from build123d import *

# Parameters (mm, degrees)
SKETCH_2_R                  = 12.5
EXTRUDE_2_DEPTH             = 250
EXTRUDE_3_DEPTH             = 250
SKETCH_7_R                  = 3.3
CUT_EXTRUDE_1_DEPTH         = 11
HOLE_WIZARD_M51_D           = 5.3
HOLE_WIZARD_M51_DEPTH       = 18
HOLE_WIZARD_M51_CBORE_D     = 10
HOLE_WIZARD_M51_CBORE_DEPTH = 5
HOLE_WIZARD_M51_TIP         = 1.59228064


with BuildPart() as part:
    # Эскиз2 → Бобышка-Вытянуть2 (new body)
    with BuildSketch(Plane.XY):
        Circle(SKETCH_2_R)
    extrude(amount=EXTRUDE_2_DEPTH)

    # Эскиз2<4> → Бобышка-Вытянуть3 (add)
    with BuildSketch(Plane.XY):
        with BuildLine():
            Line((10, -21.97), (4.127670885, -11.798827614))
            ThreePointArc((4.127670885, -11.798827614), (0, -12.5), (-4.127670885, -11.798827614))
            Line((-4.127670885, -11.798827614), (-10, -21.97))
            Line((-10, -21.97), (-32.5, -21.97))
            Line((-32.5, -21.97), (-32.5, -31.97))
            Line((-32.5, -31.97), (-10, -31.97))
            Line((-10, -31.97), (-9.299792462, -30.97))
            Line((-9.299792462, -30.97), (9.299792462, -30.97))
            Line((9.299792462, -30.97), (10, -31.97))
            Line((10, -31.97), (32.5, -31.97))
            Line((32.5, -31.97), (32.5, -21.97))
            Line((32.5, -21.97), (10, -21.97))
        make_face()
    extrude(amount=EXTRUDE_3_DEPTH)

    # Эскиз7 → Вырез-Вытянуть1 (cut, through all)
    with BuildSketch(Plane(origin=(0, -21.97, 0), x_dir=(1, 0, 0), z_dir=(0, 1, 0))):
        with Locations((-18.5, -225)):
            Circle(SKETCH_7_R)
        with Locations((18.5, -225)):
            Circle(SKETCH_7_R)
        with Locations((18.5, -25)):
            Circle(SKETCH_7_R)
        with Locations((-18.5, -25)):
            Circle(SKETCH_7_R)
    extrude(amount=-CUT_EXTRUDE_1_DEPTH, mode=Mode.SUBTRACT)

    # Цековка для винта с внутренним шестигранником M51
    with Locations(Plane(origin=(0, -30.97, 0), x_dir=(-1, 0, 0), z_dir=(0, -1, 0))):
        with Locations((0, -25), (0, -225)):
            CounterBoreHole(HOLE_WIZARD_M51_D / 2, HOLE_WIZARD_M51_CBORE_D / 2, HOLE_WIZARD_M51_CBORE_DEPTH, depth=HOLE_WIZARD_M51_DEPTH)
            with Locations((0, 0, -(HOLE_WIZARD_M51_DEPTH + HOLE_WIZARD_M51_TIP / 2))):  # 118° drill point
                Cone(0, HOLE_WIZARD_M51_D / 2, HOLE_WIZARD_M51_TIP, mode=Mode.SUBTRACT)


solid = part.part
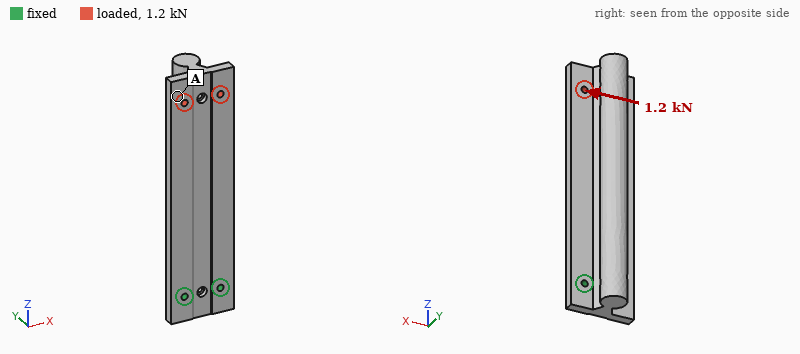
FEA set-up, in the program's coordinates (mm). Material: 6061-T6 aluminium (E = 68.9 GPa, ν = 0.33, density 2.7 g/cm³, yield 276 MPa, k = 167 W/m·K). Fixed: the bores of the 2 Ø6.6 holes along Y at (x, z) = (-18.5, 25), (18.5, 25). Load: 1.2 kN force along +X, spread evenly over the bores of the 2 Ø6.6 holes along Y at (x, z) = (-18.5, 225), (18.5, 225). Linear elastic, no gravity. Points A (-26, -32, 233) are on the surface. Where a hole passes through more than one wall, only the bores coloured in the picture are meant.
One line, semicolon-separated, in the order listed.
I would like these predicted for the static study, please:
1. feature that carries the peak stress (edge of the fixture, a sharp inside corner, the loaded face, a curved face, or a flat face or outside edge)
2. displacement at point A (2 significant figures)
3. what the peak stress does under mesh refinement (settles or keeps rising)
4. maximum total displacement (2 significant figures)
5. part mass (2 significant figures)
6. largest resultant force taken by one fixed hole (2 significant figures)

edge of the fixture; 0.24 mm; keeps rising; 0.27 mm; 840 g; 6.0 kN
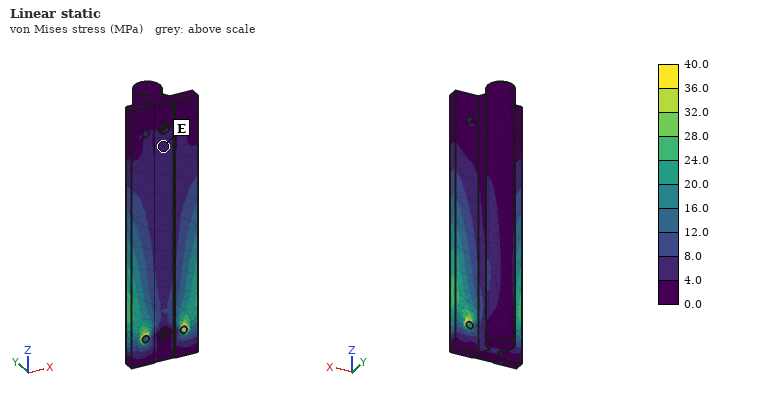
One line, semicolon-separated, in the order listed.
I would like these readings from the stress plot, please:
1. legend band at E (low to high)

4.0 to 8.0 MPa
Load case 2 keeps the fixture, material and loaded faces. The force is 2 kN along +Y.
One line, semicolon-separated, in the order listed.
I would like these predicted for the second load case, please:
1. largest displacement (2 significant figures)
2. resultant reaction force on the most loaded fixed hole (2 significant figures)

2.2 mm; 1.5 kN
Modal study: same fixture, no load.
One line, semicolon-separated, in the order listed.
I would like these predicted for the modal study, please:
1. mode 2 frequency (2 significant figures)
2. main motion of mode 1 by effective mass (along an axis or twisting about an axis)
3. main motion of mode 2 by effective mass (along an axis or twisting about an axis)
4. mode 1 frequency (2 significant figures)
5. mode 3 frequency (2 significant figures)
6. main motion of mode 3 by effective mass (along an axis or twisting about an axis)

680 Hz; along Y; along X; 290 Hz; 1400 Hz; twisting about Z
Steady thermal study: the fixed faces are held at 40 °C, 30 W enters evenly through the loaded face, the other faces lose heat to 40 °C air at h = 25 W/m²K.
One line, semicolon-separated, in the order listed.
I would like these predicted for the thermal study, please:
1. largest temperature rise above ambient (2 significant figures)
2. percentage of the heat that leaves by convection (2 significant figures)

23 K; 49 %
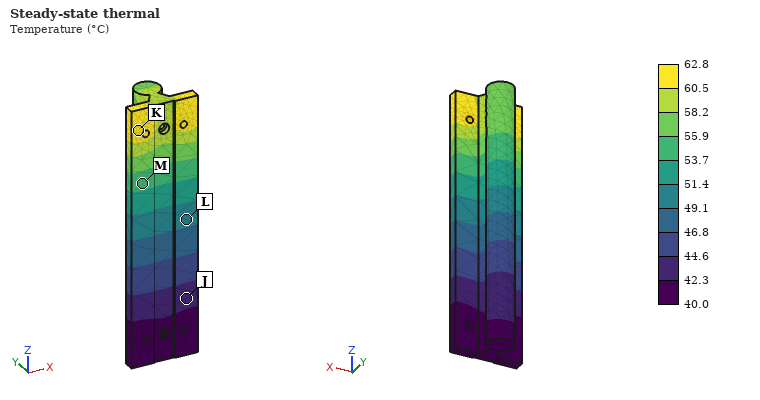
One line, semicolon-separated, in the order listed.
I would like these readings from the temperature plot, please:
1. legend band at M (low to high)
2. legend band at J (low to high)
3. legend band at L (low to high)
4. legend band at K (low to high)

53.7 to 55.9 °C; 42.3 to 44.6 °C; 49.1 to 51.4 °C; 60.5 to 62.8 °C
